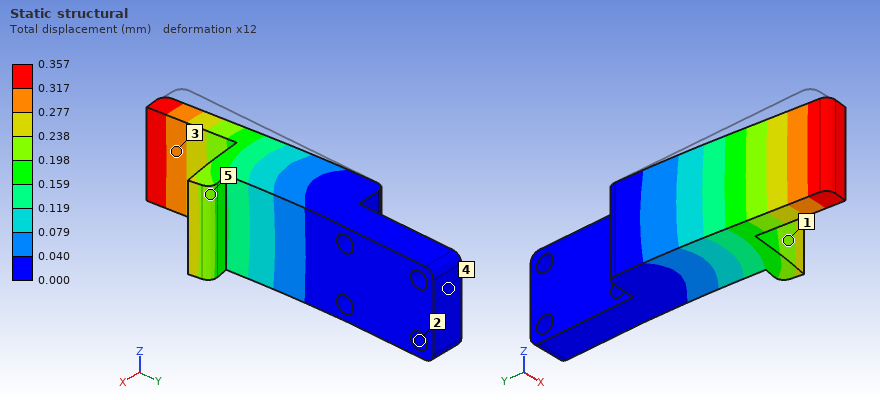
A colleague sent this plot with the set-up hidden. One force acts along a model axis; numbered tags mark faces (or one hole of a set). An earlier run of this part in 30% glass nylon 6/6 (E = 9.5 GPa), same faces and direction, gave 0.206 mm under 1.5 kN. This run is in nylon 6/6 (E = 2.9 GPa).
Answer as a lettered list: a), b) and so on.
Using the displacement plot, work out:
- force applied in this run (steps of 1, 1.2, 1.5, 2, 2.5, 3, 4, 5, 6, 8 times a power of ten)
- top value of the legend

a) 800 N
b) 0.357 mm
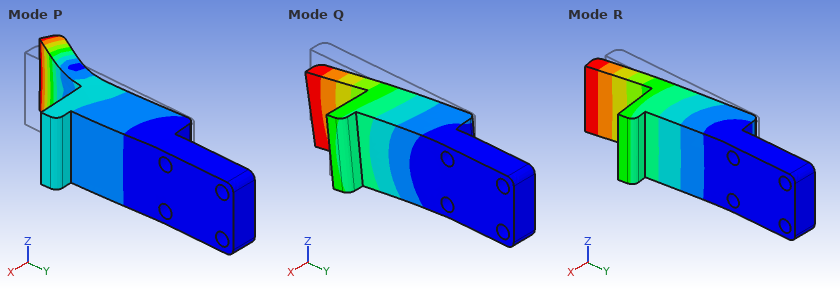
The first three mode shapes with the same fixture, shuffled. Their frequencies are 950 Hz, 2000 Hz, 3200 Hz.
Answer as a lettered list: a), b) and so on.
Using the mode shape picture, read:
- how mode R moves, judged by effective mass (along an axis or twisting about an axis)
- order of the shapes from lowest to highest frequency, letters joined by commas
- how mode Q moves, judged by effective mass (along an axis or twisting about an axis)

a) along X
b) R, Q, P
c) along Z
